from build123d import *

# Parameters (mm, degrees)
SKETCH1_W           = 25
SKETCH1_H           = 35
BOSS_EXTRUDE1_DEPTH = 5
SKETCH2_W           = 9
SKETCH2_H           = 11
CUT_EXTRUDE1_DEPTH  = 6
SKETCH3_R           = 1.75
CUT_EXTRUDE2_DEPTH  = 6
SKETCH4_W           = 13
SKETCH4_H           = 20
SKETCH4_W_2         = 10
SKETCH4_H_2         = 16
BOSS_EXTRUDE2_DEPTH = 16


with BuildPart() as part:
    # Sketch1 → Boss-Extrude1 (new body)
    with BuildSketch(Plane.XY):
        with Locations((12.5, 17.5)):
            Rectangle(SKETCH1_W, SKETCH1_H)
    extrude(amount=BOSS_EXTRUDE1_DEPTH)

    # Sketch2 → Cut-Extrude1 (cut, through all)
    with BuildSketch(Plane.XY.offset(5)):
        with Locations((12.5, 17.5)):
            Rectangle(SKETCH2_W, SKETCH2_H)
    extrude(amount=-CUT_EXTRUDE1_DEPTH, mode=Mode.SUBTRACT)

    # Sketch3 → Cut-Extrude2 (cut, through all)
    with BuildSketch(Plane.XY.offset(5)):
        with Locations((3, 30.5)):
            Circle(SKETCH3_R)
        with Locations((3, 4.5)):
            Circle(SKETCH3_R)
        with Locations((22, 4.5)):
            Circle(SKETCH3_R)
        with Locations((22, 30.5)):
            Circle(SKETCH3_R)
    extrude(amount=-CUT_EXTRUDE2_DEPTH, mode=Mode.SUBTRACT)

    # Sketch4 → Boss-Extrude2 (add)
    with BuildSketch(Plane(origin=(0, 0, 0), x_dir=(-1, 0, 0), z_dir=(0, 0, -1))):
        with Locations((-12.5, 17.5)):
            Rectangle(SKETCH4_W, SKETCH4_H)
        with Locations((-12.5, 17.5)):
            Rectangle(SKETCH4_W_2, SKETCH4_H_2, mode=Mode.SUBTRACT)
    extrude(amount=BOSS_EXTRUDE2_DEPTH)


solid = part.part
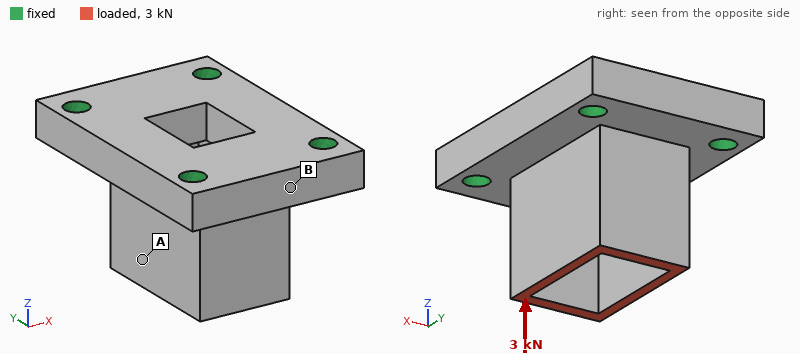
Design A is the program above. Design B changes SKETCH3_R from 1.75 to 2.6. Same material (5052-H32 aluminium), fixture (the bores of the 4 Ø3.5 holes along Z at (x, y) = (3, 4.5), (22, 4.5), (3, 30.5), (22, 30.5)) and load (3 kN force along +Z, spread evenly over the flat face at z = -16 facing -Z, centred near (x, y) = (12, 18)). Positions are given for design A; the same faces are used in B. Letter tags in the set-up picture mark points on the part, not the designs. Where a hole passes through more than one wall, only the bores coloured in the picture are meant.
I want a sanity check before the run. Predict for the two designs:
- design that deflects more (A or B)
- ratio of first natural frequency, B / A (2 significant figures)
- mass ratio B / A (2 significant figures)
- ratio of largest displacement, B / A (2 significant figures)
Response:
A
1.0
0.96
0.85
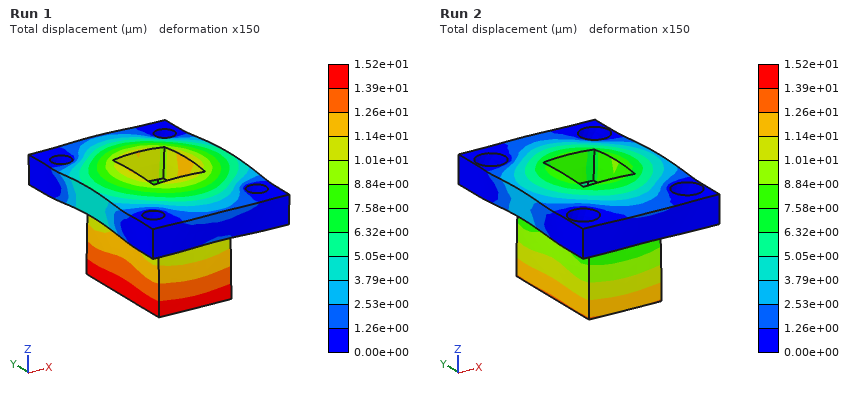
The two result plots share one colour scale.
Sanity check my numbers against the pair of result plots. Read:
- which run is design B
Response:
Run 2
